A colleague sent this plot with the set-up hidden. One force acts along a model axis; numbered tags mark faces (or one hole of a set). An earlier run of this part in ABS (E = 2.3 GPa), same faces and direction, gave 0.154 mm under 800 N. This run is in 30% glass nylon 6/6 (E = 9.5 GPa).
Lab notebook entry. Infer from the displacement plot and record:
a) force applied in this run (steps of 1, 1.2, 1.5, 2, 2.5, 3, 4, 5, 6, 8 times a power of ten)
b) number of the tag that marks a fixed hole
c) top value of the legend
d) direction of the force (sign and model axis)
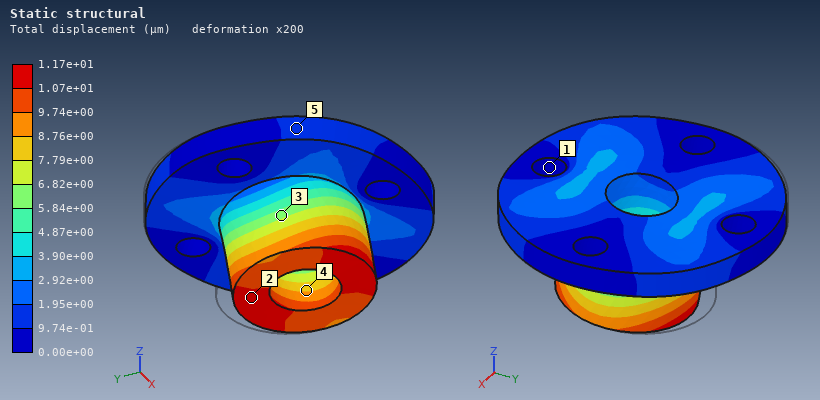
250 N
1
1.17e+01 µm
-Y
